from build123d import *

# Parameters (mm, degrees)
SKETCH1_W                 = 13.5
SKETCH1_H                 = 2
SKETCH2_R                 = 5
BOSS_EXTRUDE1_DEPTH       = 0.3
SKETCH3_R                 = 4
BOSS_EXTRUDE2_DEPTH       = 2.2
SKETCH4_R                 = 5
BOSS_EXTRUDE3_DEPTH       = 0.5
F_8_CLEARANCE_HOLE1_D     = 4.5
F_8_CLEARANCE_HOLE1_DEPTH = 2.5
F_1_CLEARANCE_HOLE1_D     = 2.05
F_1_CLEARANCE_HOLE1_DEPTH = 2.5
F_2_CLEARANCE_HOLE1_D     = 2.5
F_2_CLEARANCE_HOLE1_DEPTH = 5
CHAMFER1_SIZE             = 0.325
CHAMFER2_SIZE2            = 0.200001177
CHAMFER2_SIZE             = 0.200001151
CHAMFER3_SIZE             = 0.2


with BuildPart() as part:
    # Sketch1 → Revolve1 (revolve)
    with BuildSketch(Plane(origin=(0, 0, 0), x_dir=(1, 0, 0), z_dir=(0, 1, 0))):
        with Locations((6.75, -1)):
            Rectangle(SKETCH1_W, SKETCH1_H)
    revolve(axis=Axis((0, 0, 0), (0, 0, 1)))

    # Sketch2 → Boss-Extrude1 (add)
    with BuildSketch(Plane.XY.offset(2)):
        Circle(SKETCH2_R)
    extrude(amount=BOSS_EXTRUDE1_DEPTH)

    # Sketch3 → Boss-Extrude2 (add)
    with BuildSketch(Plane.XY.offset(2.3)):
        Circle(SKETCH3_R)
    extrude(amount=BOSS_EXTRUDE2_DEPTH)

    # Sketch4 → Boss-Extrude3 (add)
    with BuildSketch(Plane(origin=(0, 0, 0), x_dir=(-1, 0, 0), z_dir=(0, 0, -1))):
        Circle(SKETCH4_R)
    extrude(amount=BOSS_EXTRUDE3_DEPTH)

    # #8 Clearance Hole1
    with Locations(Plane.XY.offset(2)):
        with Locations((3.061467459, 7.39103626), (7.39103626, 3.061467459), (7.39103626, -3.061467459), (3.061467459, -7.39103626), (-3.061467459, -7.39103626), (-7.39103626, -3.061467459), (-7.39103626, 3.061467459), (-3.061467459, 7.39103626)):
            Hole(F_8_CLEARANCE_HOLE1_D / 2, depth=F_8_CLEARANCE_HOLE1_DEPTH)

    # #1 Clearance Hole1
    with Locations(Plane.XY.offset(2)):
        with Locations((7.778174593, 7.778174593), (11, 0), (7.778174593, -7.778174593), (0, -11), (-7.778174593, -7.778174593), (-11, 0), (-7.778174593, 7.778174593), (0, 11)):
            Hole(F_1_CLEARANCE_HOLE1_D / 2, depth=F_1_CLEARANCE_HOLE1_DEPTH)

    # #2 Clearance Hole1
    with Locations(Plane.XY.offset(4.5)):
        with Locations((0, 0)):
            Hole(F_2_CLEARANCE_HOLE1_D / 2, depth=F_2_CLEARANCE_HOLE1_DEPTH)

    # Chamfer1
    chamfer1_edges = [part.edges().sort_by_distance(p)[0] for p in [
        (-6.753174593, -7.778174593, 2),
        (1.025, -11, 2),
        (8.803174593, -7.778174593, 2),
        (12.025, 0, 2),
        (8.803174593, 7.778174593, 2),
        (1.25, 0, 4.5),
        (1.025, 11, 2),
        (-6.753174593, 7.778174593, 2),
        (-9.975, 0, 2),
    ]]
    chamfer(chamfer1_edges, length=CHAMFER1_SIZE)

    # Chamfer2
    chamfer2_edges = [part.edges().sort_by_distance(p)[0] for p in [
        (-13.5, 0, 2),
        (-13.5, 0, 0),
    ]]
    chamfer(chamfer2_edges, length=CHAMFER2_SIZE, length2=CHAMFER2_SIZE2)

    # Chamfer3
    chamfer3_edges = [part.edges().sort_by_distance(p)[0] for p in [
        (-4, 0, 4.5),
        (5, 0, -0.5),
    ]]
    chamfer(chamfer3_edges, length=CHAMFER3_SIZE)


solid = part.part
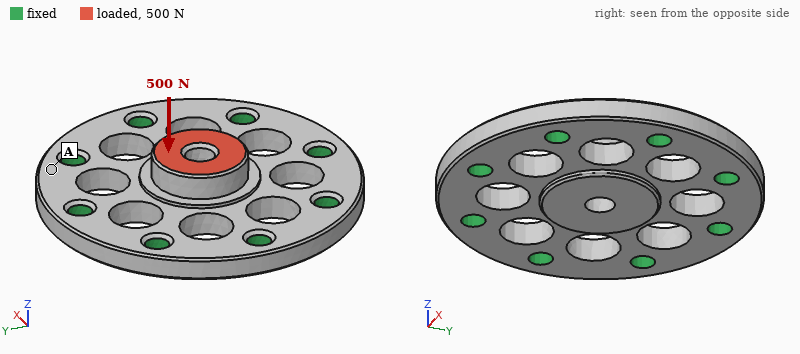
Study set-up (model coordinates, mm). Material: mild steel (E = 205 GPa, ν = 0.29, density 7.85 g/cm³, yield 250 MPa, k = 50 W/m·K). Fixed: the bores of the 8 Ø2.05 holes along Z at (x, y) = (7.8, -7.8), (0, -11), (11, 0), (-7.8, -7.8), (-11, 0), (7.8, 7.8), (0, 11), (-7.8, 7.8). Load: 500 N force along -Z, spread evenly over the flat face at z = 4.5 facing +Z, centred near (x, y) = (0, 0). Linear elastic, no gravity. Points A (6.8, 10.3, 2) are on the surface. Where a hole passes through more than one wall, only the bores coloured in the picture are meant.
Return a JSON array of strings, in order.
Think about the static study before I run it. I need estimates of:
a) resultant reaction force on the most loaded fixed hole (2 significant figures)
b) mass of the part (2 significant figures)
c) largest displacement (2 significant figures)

["65 N", "7.7 g", "5.0 µm"]
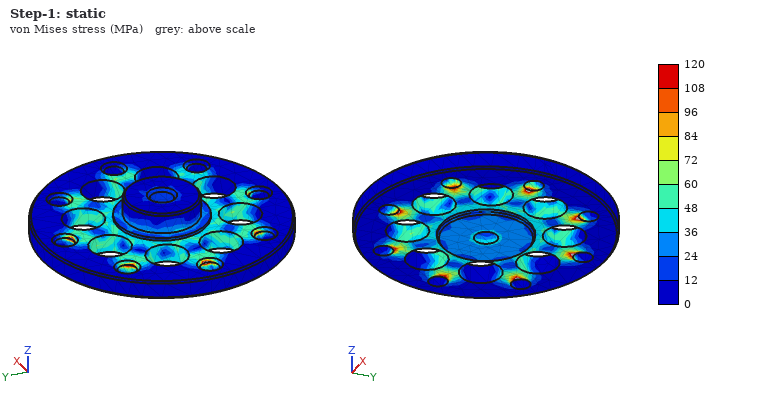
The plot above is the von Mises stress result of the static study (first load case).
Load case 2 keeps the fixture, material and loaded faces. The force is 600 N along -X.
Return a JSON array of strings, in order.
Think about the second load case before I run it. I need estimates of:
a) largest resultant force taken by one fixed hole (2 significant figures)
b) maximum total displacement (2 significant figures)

["150 N", "4.4 µm"]
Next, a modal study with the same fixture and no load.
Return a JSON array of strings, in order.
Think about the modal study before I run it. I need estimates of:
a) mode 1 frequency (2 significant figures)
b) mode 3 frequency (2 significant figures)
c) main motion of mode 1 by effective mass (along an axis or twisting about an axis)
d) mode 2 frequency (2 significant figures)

["31 kHz", "55 kHz", "along Z", "55 kHz"]
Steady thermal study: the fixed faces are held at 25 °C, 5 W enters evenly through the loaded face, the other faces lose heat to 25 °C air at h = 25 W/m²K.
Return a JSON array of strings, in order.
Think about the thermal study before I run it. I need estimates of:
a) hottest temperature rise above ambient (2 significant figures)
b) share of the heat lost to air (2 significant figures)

["23 K", "3.4 %"]
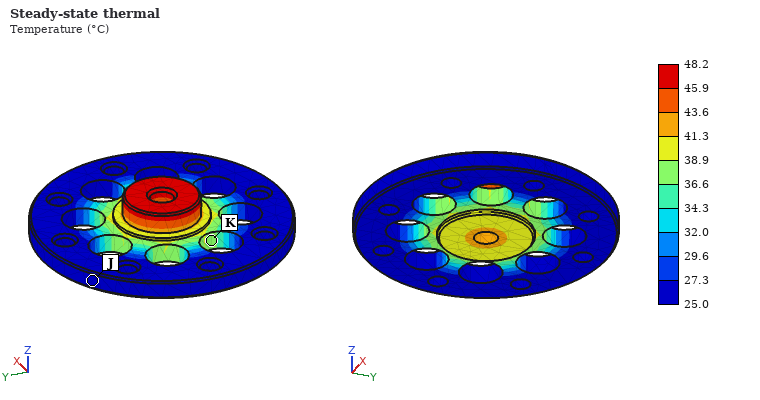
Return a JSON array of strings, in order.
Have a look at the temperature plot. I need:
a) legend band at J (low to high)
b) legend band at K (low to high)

["25.0 to 27.3 °C", "36.6 to 38.9 °C"]
